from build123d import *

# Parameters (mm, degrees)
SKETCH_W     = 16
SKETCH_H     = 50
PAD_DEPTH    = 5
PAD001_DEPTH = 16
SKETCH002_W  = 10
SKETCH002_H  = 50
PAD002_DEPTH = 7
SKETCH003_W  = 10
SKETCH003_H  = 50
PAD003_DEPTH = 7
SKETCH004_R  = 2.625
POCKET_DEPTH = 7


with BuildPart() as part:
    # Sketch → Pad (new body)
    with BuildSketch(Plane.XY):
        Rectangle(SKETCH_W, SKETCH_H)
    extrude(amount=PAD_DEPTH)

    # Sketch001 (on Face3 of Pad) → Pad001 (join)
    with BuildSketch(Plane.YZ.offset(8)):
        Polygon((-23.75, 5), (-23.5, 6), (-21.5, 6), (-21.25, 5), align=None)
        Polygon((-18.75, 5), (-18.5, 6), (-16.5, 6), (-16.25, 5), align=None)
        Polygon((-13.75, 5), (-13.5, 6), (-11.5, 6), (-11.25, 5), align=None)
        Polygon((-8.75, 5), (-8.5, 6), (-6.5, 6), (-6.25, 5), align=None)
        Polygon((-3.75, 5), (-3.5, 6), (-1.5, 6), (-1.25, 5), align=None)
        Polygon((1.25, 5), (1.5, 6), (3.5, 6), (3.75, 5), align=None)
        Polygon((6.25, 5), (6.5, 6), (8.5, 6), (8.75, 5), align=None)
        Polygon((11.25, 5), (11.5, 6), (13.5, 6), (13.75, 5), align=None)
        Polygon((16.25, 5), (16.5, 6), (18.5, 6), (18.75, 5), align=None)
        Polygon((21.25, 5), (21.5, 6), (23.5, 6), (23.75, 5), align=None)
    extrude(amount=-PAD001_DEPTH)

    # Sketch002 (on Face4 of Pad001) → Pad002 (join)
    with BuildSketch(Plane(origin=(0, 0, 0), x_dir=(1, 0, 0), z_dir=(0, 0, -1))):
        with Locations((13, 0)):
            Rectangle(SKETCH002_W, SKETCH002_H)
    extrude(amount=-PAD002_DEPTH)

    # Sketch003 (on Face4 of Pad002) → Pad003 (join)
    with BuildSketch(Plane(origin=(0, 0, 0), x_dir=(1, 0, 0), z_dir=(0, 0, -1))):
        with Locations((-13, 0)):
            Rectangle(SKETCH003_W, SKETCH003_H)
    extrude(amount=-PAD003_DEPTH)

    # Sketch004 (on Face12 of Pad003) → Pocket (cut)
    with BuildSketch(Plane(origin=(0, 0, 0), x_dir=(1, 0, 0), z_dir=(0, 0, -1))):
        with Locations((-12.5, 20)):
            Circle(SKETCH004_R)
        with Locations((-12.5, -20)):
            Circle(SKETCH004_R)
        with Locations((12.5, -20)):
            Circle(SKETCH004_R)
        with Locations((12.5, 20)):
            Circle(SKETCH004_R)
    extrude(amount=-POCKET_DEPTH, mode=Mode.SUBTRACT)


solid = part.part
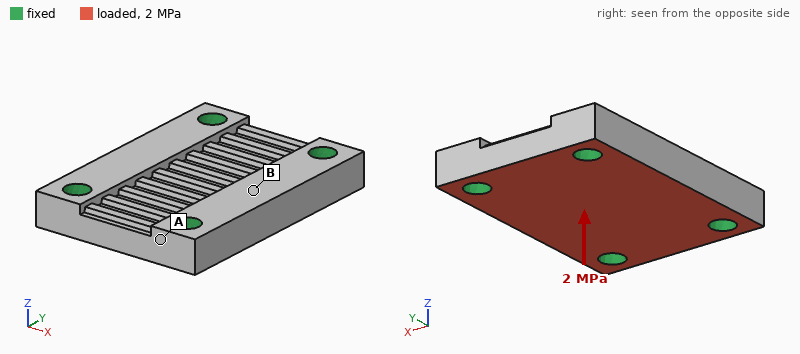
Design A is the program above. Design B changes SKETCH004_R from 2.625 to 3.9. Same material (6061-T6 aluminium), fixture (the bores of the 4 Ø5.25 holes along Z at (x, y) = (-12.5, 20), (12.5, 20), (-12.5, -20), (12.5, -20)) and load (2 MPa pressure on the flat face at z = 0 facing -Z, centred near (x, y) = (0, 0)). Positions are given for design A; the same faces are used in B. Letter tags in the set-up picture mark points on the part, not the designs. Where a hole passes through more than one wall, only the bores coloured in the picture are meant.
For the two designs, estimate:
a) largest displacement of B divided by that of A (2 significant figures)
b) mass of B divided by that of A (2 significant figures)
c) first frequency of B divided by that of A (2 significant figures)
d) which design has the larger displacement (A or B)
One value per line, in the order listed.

0.77
0.93
1.2
A
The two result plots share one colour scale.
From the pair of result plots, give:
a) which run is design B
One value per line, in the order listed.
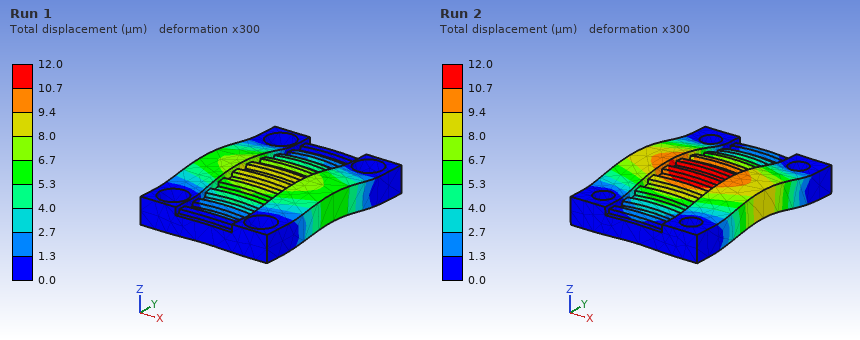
Run 1
